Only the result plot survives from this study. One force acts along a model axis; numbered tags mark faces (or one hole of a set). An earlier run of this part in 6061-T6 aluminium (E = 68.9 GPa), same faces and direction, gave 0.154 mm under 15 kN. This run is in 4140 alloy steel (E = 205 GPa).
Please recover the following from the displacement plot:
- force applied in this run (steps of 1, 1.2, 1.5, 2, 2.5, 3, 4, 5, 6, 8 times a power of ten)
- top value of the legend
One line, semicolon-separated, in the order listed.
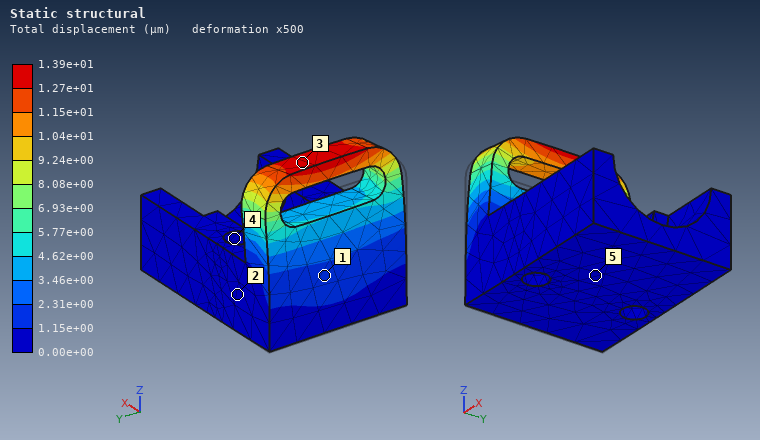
4 kN; 1.39e+01 µm
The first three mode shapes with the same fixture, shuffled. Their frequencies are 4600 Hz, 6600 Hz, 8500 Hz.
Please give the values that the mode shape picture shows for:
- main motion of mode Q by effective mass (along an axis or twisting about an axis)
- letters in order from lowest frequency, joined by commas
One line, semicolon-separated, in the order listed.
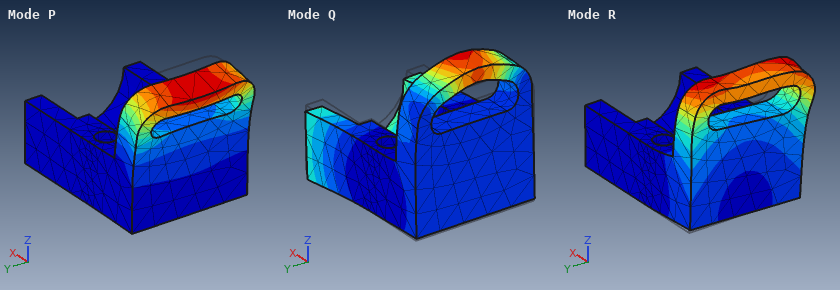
twisting about Y; P, R, Q
